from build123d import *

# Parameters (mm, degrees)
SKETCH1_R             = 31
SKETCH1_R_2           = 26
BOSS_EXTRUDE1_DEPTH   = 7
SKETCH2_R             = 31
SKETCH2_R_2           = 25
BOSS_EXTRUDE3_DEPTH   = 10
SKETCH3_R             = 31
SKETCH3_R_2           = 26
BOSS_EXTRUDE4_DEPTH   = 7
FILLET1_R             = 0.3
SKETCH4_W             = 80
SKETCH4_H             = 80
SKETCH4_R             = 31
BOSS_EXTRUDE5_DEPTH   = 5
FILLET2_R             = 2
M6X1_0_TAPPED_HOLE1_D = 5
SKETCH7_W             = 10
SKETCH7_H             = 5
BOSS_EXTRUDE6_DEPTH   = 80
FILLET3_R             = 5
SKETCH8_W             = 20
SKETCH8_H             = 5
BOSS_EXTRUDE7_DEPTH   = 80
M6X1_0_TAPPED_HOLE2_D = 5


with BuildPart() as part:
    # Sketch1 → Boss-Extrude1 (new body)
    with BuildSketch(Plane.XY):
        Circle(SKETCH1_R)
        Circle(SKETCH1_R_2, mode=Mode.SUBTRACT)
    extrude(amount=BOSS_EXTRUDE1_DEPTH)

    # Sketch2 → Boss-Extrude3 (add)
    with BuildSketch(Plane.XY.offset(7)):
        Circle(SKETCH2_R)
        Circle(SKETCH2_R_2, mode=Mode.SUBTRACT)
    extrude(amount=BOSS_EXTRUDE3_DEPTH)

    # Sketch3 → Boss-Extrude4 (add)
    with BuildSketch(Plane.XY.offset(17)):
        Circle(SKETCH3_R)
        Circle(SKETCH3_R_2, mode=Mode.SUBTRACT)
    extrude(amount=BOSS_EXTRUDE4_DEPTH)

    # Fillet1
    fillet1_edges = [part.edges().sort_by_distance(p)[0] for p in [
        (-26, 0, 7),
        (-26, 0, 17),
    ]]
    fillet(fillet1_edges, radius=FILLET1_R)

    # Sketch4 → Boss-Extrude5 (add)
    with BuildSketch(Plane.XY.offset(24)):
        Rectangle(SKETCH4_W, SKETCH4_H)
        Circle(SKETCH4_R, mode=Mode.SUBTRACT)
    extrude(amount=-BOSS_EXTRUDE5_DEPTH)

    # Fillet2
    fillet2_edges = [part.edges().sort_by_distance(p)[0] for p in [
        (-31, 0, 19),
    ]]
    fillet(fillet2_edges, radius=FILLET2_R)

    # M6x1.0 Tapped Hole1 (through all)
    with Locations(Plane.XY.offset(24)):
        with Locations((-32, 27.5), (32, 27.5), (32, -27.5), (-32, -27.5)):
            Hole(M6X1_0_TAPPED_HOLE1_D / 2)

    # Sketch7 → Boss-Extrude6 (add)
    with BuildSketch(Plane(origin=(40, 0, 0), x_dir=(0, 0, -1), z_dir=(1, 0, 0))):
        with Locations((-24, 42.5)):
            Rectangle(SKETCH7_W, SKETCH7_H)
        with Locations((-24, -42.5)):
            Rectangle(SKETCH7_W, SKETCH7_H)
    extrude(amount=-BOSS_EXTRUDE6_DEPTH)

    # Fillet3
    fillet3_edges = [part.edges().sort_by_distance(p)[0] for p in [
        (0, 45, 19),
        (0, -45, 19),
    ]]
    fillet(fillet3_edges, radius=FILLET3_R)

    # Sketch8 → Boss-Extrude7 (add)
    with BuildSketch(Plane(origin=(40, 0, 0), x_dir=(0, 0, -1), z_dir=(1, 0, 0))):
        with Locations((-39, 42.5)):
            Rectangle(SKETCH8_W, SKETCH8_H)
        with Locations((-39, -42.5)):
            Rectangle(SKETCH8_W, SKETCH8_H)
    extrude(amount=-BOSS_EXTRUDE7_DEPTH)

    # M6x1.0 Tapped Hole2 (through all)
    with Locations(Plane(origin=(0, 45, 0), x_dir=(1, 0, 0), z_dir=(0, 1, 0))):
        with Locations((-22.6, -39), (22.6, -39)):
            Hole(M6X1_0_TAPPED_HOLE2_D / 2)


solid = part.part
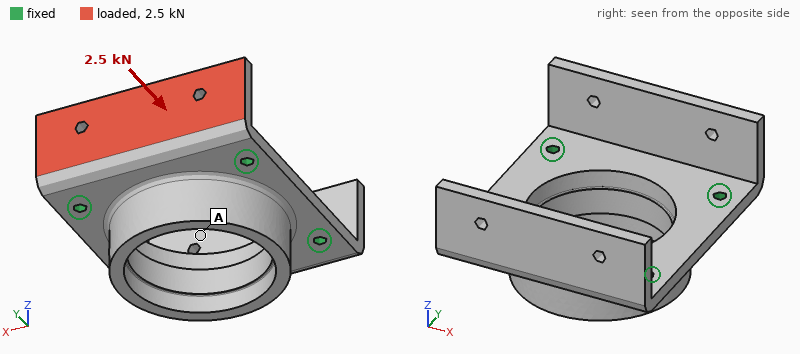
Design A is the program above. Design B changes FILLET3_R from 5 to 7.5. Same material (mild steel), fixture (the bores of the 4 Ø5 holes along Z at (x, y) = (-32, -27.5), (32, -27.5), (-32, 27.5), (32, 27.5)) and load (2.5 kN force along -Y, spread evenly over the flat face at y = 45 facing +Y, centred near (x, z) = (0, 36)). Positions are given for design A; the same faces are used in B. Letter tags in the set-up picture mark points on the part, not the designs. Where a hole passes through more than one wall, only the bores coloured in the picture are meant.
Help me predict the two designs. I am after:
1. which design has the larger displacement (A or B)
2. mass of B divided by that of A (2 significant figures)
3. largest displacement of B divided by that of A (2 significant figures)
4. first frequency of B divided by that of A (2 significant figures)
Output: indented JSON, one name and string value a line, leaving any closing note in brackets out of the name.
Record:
{
  "which design has the larger displacement": "B",
  "mass of B divided by that of A": "0.98",
  "largest displacement of B divided by that of A": "1.1",
  "first frequency of B divided by that of A": "0.98"
}
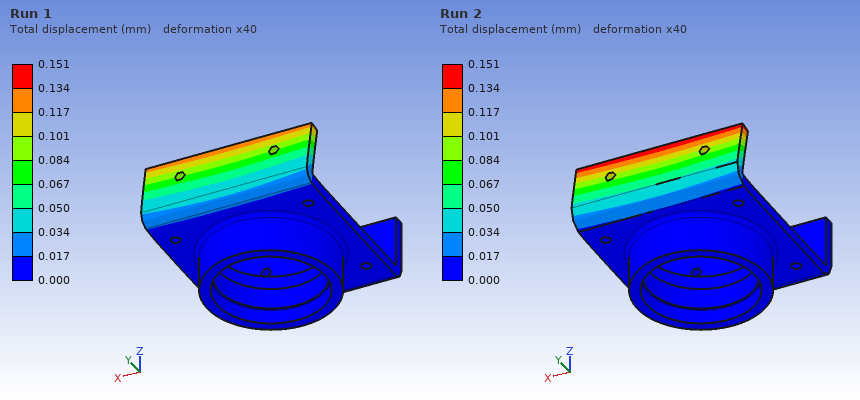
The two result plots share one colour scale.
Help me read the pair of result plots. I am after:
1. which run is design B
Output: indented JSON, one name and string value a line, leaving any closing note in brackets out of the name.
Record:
{
  "which run is design B": "Run 2"
}
